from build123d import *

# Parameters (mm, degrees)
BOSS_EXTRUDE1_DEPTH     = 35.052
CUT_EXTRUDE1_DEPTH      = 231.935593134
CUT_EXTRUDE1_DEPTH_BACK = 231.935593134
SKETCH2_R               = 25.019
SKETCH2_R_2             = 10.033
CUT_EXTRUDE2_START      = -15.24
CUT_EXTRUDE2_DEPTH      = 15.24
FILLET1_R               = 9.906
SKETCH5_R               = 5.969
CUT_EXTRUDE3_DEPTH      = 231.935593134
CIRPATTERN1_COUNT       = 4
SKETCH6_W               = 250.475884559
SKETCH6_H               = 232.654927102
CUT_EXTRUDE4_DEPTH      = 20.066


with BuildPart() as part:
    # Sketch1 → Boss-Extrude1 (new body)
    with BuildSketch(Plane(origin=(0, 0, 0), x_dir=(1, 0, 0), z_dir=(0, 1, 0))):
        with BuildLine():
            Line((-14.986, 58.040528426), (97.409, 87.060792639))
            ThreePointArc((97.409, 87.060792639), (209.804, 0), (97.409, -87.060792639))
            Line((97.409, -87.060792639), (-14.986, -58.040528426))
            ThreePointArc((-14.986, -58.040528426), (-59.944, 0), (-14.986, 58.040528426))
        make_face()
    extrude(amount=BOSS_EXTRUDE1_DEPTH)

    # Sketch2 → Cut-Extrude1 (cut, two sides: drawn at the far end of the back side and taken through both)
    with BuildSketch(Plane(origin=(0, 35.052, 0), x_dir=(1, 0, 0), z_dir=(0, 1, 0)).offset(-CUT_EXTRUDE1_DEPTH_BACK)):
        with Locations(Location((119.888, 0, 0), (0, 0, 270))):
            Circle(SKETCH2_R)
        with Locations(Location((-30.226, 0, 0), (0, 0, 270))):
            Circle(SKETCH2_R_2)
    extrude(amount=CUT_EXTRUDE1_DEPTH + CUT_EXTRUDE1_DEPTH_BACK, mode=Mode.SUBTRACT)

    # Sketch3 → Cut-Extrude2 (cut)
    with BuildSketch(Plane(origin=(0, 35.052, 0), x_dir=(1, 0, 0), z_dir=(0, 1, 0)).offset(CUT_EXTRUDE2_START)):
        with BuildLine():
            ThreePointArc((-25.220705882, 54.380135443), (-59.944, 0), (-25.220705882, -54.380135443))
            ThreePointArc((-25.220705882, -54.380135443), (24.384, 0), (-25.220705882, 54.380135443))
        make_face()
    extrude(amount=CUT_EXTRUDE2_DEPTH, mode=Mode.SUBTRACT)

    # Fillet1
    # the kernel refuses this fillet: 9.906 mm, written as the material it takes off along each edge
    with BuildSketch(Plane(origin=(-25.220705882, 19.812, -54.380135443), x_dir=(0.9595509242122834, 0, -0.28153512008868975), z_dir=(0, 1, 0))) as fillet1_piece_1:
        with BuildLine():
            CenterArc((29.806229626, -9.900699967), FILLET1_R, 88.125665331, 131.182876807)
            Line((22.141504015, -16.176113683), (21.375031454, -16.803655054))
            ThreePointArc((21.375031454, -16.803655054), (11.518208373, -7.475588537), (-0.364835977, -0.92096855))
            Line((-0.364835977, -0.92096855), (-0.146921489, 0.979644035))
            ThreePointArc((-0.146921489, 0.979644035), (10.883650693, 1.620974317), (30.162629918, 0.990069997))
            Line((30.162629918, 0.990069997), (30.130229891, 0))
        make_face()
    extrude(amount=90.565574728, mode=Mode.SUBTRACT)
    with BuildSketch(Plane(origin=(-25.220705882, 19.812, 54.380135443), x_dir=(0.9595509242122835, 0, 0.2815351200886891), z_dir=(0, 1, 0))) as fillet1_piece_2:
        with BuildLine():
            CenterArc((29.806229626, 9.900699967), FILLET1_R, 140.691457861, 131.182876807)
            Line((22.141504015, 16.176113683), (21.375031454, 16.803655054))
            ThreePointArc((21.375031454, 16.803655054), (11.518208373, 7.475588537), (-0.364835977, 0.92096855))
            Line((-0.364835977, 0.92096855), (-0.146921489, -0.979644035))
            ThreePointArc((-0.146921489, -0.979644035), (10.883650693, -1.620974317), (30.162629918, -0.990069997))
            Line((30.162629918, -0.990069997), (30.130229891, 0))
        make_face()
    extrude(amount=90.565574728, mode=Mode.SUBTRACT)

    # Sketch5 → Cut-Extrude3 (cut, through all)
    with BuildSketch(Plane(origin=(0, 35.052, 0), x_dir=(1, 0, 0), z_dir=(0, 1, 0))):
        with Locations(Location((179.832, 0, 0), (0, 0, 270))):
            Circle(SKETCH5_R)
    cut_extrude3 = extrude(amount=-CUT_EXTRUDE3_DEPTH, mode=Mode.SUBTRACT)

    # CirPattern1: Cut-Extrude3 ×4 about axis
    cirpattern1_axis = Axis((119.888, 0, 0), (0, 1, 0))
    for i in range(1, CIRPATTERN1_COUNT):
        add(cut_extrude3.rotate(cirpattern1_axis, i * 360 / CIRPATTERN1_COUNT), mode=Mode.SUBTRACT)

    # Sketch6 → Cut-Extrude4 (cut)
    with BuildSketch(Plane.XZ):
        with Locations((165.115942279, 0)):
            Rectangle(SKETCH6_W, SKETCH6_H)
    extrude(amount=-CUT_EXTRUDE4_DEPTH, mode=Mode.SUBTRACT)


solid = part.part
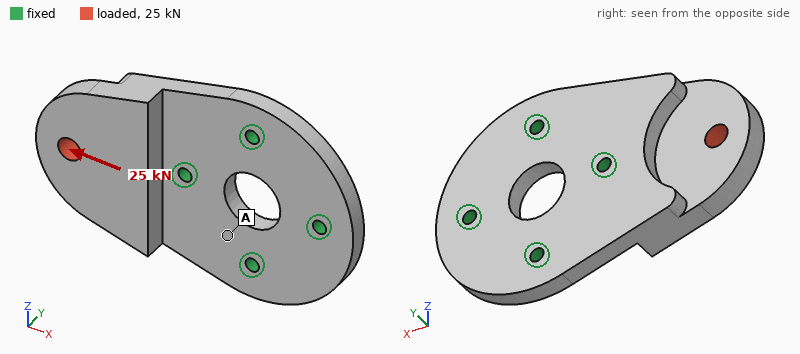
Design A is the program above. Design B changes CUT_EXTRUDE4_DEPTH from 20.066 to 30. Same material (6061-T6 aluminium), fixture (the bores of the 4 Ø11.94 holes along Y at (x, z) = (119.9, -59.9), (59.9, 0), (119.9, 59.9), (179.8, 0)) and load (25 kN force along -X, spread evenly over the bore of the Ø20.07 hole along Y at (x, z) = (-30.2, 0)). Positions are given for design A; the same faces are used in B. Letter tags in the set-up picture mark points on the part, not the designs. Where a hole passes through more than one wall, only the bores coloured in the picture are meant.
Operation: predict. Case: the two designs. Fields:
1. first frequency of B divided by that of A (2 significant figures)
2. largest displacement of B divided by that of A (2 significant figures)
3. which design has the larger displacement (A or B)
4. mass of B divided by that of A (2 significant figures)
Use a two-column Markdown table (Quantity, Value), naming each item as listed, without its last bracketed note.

| Quantity | Value |
|---|---|
| first frequency of B divided by that of A | 0.24 |
| largest displacement of B divided by that of A | 24 |
| which design has the larger displacement | B |
| mass of B divided by that of A | 0.63 |
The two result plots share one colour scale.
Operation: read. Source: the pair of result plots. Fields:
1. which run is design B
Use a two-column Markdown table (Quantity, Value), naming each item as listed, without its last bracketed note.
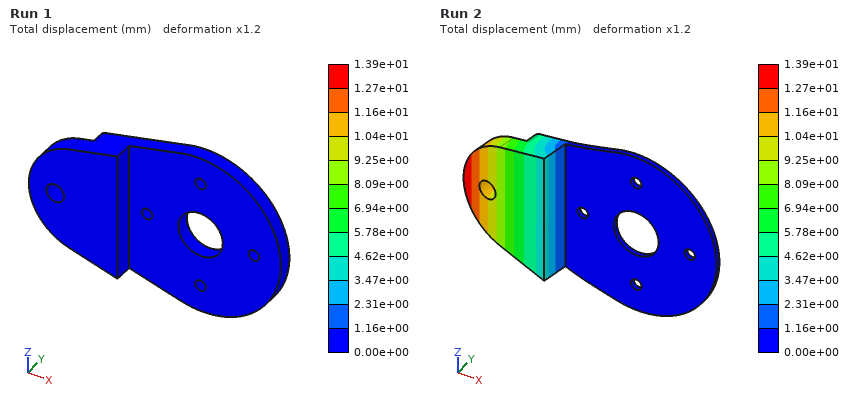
| Quantity | Value |
|---|---|
| which run is design B | Run 2 |
